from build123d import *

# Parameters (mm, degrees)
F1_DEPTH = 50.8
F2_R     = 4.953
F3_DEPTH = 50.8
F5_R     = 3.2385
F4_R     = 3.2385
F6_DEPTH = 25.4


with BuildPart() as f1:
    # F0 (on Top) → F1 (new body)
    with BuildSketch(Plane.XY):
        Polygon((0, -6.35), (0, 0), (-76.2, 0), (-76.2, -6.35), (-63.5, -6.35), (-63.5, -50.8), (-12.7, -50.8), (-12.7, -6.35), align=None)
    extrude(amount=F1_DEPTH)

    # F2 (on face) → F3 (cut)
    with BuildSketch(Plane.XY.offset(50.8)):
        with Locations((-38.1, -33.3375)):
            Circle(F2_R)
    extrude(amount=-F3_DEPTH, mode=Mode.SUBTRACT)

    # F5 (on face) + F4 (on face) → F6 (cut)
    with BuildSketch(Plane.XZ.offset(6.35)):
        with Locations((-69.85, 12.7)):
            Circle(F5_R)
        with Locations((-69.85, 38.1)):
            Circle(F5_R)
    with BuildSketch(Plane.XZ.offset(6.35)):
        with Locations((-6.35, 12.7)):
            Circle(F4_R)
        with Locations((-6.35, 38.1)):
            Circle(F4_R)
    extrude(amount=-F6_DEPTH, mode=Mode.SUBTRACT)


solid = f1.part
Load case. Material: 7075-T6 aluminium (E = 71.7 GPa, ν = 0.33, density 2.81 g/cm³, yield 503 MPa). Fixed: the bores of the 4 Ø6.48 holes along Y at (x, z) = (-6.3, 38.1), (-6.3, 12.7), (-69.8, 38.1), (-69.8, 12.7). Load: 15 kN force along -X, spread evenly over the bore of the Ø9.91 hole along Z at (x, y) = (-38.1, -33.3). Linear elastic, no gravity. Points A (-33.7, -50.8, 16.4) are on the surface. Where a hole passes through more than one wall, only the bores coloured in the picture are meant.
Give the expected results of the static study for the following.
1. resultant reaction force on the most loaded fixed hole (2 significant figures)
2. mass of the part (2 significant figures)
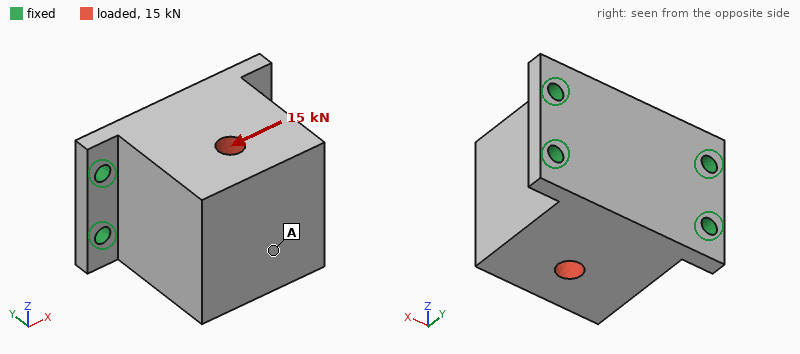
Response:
5.6 kN
380 g
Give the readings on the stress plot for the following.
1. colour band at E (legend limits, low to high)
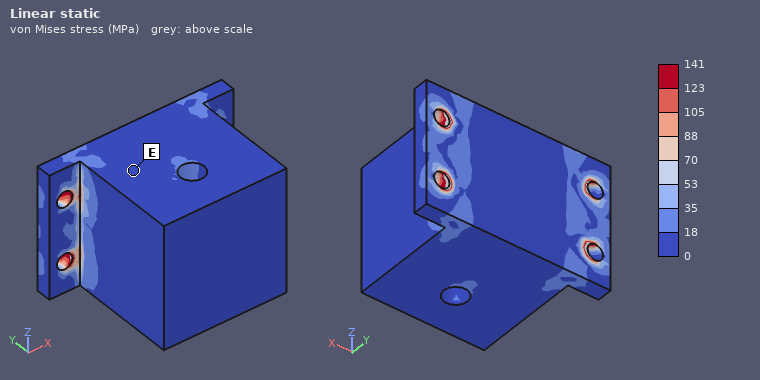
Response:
0 to 18 MPa
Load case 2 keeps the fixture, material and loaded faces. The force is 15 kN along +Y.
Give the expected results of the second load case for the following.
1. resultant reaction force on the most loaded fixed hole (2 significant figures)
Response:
4.2 kN
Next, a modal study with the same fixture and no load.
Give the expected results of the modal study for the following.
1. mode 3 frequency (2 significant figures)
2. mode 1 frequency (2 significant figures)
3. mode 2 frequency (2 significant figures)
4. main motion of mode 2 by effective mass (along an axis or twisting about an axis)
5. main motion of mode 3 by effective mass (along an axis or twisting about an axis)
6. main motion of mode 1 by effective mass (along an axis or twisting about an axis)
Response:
7600 Hz
3400 Hz
6500 Hz
along X
along Y
along Z
